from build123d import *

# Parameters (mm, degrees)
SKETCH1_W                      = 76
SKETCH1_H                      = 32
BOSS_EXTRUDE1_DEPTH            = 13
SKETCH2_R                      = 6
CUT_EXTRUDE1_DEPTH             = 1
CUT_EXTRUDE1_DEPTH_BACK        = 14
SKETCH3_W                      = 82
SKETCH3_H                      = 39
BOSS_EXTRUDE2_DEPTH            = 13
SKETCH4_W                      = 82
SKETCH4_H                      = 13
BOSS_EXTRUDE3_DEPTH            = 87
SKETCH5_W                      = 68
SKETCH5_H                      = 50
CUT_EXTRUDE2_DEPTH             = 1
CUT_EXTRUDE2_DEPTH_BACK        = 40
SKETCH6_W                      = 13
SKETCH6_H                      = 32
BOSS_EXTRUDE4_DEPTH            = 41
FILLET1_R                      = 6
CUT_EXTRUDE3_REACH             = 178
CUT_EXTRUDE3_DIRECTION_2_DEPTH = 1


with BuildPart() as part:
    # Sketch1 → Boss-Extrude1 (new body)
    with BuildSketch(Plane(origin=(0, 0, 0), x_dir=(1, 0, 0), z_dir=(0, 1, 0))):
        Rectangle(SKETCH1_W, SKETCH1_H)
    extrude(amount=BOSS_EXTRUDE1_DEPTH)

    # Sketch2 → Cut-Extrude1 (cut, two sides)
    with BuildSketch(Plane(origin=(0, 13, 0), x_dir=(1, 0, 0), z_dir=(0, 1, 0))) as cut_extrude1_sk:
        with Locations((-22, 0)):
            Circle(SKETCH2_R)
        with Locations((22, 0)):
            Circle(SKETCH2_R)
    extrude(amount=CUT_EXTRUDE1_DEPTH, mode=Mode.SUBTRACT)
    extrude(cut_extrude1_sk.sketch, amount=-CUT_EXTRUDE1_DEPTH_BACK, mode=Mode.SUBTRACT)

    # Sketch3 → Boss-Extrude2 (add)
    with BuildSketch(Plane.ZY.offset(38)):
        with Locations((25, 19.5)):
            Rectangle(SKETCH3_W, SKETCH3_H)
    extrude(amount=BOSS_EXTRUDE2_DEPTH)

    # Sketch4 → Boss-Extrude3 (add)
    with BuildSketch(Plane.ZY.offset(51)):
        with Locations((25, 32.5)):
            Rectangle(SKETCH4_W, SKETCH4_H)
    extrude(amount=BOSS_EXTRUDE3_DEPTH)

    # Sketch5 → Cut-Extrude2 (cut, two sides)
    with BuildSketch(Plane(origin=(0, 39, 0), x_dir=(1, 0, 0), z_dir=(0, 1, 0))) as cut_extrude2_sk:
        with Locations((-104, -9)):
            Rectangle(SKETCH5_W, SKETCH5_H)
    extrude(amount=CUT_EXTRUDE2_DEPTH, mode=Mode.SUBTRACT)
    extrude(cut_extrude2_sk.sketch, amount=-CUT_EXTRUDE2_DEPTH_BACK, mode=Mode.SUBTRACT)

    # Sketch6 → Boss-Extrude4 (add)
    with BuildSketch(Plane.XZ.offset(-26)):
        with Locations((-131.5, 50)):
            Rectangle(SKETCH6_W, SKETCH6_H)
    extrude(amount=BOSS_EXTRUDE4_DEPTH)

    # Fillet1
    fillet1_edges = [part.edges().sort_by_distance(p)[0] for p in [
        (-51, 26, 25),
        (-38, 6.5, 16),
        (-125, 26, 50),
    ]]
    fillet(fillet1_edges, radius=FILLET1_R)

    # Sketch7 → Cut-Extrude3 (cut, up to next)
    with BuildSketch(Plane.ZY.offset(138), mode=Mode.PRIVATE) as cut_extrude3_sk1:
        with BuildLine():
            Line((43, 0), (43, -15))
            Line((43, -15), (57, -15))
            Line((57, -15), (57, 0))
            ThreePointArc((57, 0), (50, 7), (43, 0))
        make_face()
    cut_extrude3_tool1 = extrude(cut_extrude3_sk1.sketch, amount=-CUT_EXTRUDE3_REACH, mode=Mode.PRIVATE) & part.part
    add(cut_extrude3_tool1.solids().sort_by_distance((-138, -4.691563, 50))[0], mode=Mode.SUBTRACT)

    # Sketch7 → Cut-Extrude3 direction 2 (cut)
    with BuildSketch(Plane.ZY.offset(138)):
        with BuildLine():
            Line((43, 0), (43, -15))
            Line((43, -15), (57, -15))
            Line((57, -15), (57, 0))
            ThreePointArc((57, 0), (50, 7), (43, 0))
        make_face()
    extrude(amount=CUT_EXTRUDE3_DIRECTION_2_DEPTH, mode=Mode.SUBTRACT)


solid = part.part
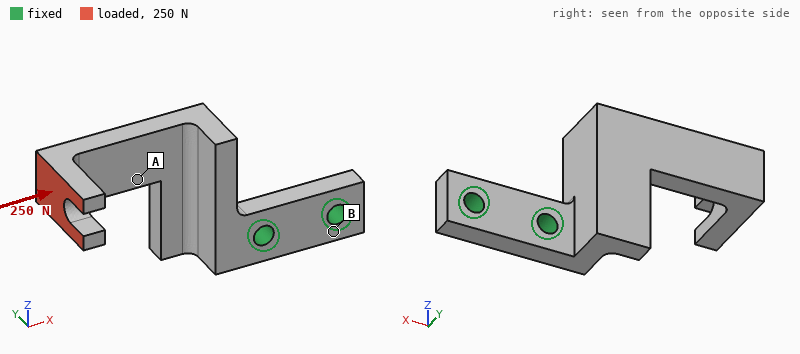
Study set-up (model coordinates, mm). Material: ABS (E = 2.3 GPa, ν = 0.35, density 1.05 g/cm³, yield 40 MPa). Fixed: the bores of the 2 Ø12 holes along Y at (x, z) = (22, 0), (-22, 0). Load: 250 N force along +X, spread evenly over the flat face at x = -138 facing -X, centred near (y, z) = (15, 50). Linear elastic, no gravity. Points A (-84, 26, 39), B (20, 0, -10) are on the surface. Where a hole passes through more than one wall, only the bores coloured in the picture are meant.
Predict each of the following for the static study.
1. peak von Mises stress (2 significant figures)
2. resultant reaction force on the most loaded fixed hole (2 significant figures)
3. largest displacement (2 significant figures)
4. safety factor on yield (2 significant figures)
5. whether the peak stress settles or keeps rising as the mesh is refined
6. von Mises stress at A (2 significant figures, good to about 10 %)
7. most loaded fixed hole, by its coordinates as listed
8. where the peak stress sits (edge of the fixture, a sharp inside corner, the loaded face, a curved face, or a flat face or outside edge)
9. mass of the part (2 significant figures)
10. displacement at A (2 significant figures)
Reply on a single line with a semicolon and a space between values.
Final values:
21 MPa; 260 N; 2.2 mm; 1.9; settles; 5.5 MPa; (-22, 0); a curved face; 140 g; 0.67 mm
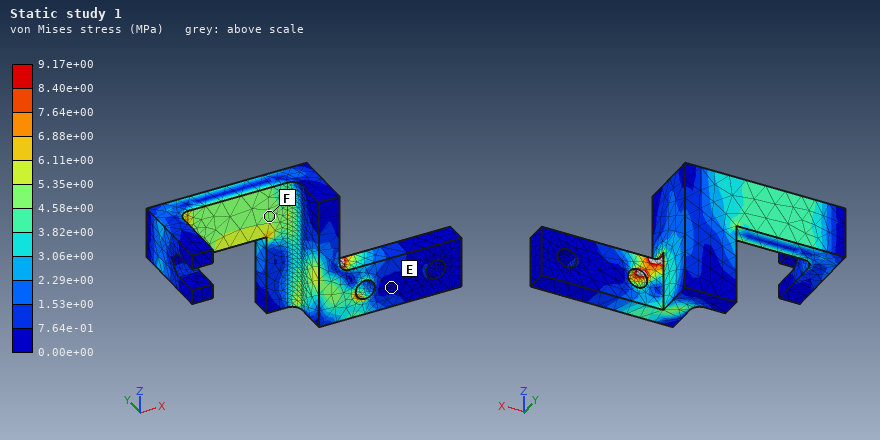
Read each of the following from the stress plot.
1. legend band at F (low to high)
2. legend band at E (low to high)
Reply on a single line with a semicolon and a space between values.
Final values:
4.58e+00 to 5.35e+00 MPa; 0.00e+00 to 7.64e-01 MPa
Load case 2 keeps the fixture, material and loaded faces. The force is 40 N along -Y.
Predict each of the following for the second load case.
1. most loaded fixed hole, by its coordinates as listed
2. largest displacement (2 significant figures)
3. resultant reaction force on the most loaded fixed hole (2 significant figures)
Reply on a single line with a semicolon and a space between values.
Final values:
(-22, 0); 2.0 mm; 50 N
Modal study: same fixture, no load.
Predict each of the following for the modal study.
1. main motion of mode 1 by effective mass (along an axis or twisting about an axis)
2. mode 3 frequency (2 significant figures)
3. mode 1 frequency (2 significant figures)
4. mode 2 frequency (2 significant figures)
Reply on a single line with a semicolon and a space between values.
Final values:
along Y; 440 Hz; 140 Hz; 230 Hz
